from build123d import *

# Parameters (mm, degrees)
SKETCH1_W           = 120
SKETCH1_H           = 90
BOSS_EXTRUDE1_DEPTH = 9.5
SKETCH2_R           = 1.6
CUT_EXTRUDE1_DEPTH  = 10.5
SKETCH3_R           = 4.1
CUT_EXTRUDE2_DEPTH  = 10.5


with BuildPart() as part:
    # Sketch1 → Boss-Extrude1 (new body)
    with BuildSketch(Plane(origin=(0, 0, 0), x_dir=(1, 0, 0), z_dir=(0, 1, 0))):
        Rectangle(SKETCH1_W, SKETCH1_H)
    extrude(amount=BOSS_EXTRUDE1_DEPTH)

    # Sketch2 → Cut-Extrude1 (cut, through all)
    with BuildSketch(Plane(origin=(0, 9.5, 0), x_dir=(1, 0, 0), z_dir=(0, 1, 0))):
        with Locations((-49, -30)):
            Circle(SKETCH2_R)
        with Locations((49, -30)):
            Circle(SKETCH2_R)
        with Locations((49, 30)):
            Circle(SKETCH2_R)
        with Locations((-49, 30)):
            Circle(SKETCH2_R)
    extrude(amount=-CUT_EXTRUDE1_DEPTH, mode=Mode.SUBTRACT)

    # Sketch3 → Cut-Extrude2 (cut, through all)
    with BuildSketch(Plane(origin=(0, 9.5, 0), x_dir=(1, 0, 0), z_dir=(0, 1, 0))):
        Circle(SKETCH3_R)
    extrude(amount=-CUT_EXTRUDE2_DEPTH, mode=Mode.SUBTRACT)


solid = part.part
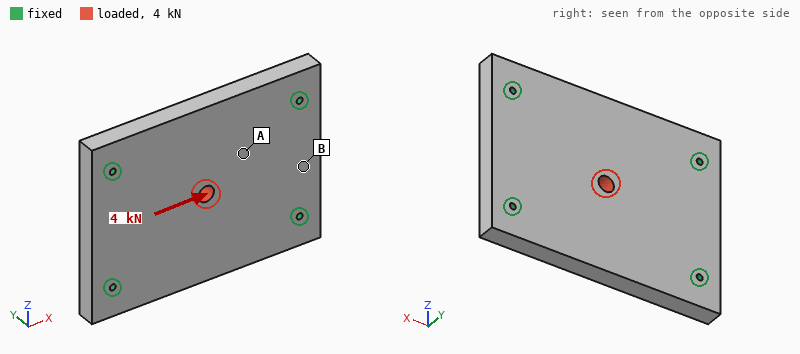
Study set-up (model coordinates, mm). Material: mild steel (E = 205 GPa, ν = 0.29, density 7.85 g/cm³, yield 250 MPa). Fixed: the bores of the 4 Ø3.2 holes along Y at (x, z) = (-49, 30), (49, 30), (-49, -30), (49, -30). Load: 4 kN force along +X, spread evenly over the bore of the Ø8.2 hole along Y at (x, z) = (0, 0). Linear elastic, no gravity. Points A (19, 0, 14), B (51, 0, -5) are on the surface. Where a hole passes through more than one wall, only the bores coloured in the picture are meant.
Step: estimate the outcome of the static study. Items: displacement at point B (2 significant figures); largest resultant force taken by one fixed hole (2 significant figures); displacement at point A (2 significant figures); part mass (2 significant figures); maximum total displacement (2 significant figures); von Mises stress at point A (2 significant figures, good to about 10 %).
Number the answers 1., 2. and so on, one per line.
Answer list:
1. 0.71 µm
2. 1.0 kN
3. 0.90 µm
4. 800 g
5. 1.9 µm
6. 4.8 MPa
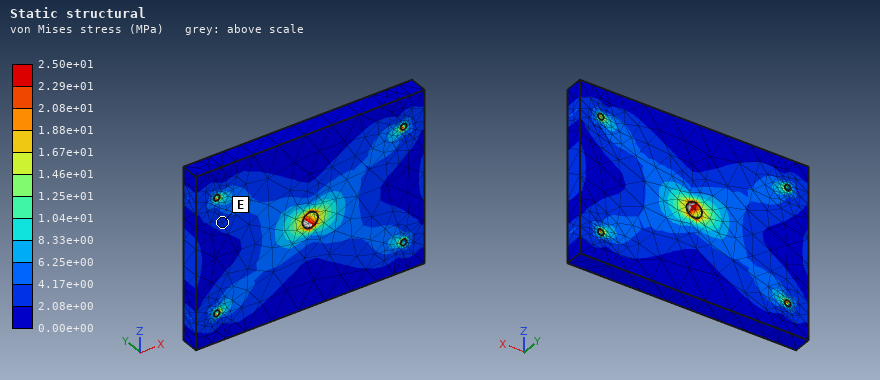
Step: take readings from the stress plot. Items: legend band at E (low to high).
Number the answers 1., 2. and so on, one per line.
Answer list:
1. 2.08e+00 to 4.17e+00 MPa
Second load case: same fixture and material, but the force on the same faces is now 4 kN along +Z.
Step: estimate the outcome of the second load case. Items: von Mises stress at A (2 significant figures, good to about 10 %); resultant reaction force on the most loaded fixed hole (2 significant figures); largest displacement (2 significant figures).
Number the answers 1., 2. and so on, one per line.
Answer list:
1. 5.8 MPa
2. 1.2 kN
3. 2.7 µm
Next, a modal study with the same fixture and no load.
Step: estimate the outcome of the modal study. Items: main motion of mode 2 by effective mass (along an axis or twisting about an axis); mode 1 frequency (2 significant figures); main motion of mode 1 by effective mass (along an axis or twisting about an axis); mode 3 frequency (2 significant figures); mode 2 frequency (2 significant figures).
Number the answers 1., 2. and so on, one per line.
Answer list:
1. twisting about X
2. 3700 Hz
3. along Y
4. 8100 Hz
5. 5200 Hz
